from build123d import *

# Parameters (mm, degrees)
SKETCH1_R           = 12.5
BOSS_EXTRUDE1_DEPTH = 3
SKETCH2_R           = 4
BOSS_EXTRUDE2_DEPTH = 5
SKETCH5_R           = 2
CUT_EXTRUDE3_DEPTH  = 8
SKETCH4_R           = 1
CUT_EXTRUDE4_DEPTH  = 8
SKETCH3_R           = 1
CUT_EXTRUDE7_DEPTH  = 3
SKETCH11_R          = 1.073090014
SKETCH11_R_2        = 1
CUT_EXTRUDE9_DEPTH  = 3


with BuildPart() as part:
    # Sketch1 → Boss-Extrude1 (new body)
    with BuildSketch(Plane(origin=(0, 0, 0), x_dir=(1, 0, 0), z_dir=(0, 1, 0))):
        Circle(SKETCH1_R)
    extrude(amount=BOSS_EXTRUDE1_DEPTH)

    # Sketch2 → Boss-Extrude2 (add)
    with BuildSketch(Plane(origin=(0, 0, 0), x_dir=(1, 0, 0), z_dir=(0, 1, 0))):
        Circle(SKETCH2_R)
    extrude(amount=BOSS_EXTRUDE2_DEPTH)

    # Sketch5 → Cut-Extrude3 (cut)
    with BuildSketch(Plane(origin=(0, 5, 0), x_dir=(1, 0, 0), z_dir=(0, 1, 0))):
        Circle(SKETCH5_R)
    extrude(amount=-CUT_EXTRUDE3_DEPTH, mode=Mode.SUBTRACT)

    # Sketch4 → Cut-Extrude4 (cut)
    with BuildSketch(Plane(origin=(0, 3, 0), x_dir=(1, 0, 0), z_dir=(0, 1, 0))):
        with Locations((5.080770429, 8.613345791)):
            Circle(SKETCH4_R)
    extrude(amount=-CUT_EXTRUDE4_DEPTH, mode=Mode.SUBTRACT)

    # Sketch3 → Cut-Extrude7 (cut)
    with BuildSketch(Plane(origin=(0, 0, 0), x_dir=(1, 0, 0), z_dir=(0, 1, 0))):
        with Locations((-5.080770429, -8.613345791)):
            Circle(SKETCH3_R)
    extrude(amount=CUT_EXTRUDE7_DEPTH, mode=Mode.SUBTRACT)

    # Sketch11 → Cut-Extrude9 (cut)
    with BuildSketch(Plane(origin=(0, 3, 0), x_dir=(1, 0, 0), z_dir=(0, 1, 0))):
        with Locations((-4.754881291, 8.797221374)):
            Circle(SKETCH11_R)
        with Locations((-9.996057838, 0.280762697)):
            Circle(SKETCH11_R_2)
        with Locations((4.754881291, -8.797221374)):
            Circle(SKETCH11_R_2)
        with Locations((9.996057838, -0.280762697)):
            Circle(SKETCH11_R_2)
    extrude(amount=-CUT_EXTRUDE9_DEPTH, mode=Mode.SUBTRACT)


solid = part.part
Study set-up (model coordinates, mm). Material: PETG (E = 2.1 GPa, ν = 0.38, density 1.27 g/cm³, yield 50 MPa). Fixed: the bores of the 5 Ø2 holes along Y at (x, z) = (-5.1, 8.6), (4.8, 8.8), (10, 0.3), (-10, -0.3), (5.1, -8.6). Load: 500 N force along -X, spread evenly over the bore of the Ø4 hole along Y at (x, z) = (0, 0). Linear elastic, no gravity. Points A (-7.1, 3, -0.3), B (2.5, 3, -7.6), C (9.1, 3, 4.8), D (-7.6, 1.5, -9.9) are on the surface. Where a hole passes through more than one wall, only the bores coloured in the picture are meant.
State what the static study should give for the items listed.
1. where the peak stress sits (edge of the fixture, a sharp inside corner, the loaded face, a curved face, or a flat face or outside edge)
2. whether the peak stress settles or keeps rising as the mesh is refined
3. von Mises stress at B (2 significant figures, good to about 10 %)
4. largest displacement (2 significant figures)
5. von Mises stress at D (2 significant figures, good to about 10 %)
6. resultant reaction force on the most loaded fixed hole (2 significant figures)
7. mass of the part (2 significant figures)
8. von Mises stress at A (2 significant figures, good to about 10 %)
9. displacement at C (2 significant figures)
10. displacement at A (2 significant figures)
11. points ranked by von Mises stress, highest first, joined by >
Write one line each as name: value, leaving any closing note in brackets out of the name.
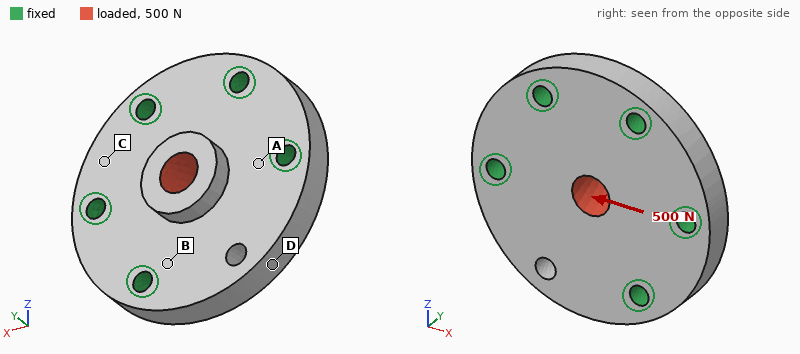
where the peak stress sits: edge of the fixture
whether the peak stress settles or keeps rising as the mesh is refined: keeps rising
von Mises stress at B: 5.6 MPa
largest displacement: 66 µm
von Mises stress at D: 3.3 MPa
resultant reaction force on the most loaded fixed hole: 150 N
mass of the part: 1.8 g
von Mises stress at A: 12 MPa
displacement at C: 11 µm
displacement at A: 10 µm
points ranked by von Mises stress, highest first, joined by >: A > B > D > C
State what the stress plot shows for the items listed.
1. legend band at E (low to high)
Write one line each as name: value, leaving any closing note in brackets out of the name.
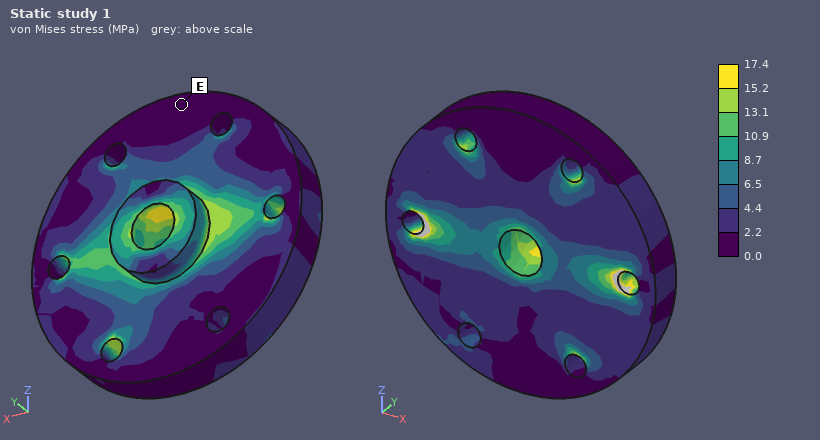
legend band at E: 0.0 to 2.2 MPa
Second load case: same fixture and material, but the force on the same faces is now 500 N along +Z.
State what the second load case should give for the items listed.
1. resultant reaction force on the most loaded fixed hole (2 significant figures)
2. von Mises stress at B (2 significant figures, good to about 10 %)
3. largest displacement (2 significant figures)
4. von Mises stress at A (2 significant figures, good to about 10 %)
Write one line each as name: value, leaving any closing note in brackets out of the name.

resultant reaction force on the most loaded fixed hole: 140 N
von Mises stress at B: 7.0 MPa
largest displacement: 72 µm
von Mises stress at A: 4.5 MPa
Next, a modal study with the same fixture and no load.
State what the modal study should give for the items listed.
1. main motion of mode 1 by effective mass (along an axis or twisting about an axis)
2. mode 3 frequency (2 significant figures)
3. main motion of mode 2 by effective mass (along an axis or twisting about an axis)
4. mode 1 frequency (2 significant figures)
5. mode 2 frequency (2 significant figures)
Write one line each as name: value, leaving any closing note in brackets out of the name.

main motion of mode 1 by effective mass: along Y
mode 3 frequency: 19 kHz
main motion of mode 2 by effective mass: along Y
mode 1 frequency: 8500 Hz
mode 2 frequency: 14 kHz
